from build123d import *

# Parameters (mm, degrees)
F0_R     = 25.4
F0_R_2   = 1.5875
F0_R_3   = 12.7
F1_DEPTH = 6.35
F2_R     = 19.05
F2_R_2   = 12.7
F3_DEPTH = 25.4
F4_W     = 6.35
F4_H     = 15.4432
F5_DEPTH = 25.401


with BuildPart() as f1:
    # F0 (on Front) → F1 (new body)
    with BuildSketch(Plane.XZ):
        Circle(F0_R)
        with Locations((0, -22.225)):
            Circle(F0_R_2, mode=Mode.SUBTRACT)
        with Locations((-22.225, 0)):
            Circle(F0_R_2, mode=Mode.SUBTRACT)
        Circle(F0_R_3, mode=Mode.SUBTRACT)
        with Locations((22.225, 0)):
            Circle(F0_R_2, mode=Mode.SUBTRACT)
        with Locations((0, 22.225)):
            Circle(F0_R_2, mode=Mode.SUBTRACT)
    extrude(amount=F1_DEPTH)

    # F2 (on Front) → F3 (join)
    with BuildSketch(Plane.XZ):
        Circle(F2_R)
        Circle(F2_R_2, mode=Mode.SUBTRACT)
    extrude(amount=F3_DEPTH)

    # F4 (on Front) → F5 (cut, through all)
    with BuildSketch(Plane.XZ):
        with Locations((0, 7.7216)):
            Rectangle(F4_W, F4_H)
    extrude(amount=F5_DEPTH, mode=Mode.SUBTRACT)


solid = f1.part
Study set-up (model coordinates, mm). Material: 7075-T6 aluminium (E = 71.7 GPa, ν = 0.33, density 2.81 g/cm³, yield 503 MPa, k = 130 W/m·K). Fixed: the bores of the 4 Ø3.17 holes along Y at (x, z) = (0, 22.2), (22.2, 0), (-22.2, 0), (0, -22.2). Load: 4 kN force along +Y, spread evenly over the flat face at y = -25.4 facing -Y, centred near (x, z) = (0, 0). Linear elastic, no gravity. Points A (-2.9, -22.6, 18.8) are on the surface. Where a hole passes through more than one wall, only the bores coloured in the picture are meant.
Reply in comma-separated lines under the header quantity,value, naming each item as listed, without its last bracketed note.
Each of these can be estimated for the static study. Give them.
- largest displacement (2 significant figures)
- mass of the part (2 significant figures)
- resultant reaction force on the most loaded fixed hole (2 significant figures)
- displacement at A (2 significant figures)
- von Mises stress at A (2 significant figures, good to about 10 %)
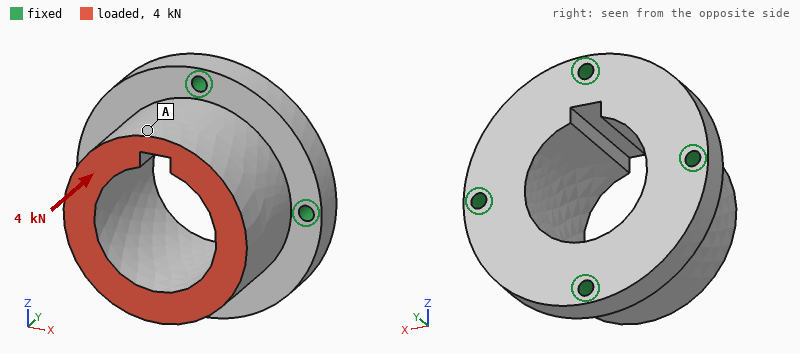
quantity,value
largest displacement,6.1 µm
mass of the part,59 g
resultant reaction force on the most loaded fixed hole,1.1 kN
displacement at A,5.5 µm
von Mises stress at A,6.6 MPa
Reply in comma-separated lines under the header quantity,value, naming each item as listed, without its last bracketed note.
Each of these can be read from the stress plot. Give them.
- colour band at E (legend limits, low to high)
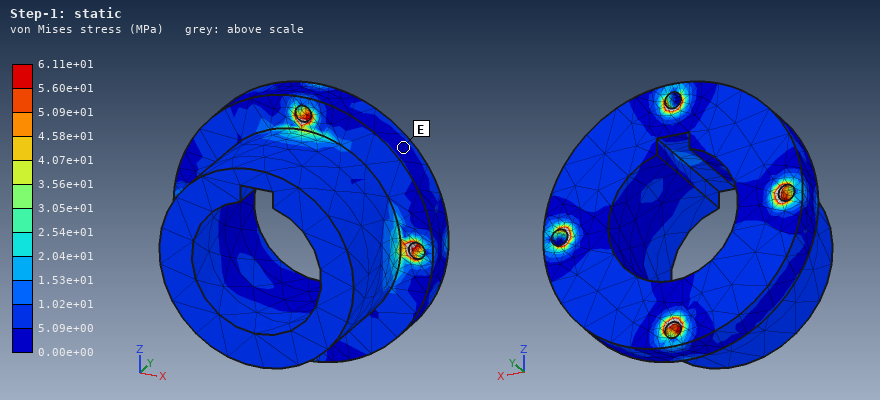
quantity,value
colour band at E,0.00e+00 to 5.09e+00 MPa
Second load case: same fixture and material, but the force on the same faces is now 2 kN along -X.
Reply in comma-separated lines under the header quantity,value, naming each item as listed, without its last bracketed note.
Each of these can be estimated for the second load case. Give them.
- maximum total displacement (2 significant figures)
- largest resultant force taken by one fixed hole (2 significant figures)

quantity,value
maximum total displacement,14 µm
largest resultant force taken by one fixed hole,1.2 kN
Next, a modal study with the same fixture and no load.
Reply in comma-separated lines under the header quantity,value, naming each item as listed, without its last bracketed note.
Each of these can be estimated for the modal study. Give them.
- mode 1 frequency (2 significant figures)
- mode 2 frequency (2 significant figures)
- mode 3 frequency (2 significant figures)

quantity,value
mode 1 frequency,16 kHz
mode 2 frequency,16 kHz
mode 3 frequency,17 kHz
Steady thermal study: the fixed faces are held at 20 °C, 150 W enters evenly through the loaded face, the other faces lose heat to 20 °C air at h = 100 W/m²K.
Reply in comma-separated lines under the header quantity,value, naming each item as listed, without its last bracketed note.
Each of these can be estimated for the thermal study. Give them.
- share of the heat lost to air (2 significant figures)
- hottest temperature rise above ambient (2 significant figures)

quantity,value
share of the heat lost to air,12 %
hottest temperature rise above ambient,53 K
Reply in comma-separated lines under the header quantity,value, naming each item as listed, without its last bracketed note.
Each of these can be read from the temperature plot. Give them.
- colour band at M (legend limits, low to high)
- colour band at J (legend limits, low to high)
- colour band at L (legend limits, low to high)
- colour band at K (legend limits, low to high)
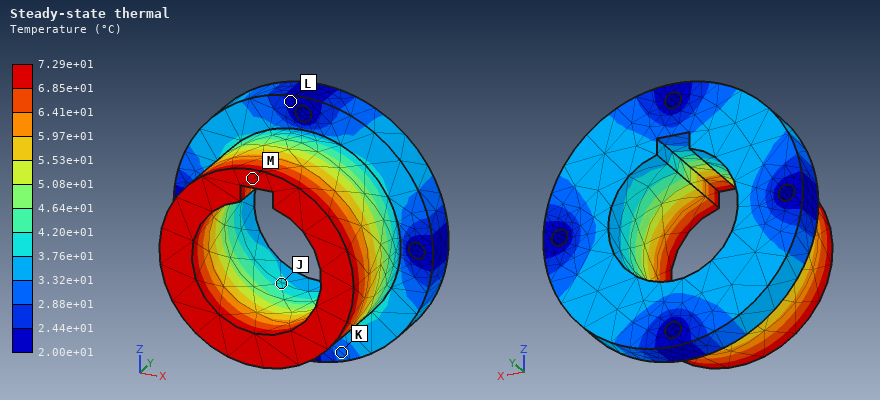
quantity,value
colour band at M,6.85e+01 to 7.29e+01 °C
colour band at J,3.76e+01 to 4.20e+01 °C
colour band at L,2.00e+01 to 2.44e+01 °C
colour band at K,2.88e+01 to 3.32e+01 °C
